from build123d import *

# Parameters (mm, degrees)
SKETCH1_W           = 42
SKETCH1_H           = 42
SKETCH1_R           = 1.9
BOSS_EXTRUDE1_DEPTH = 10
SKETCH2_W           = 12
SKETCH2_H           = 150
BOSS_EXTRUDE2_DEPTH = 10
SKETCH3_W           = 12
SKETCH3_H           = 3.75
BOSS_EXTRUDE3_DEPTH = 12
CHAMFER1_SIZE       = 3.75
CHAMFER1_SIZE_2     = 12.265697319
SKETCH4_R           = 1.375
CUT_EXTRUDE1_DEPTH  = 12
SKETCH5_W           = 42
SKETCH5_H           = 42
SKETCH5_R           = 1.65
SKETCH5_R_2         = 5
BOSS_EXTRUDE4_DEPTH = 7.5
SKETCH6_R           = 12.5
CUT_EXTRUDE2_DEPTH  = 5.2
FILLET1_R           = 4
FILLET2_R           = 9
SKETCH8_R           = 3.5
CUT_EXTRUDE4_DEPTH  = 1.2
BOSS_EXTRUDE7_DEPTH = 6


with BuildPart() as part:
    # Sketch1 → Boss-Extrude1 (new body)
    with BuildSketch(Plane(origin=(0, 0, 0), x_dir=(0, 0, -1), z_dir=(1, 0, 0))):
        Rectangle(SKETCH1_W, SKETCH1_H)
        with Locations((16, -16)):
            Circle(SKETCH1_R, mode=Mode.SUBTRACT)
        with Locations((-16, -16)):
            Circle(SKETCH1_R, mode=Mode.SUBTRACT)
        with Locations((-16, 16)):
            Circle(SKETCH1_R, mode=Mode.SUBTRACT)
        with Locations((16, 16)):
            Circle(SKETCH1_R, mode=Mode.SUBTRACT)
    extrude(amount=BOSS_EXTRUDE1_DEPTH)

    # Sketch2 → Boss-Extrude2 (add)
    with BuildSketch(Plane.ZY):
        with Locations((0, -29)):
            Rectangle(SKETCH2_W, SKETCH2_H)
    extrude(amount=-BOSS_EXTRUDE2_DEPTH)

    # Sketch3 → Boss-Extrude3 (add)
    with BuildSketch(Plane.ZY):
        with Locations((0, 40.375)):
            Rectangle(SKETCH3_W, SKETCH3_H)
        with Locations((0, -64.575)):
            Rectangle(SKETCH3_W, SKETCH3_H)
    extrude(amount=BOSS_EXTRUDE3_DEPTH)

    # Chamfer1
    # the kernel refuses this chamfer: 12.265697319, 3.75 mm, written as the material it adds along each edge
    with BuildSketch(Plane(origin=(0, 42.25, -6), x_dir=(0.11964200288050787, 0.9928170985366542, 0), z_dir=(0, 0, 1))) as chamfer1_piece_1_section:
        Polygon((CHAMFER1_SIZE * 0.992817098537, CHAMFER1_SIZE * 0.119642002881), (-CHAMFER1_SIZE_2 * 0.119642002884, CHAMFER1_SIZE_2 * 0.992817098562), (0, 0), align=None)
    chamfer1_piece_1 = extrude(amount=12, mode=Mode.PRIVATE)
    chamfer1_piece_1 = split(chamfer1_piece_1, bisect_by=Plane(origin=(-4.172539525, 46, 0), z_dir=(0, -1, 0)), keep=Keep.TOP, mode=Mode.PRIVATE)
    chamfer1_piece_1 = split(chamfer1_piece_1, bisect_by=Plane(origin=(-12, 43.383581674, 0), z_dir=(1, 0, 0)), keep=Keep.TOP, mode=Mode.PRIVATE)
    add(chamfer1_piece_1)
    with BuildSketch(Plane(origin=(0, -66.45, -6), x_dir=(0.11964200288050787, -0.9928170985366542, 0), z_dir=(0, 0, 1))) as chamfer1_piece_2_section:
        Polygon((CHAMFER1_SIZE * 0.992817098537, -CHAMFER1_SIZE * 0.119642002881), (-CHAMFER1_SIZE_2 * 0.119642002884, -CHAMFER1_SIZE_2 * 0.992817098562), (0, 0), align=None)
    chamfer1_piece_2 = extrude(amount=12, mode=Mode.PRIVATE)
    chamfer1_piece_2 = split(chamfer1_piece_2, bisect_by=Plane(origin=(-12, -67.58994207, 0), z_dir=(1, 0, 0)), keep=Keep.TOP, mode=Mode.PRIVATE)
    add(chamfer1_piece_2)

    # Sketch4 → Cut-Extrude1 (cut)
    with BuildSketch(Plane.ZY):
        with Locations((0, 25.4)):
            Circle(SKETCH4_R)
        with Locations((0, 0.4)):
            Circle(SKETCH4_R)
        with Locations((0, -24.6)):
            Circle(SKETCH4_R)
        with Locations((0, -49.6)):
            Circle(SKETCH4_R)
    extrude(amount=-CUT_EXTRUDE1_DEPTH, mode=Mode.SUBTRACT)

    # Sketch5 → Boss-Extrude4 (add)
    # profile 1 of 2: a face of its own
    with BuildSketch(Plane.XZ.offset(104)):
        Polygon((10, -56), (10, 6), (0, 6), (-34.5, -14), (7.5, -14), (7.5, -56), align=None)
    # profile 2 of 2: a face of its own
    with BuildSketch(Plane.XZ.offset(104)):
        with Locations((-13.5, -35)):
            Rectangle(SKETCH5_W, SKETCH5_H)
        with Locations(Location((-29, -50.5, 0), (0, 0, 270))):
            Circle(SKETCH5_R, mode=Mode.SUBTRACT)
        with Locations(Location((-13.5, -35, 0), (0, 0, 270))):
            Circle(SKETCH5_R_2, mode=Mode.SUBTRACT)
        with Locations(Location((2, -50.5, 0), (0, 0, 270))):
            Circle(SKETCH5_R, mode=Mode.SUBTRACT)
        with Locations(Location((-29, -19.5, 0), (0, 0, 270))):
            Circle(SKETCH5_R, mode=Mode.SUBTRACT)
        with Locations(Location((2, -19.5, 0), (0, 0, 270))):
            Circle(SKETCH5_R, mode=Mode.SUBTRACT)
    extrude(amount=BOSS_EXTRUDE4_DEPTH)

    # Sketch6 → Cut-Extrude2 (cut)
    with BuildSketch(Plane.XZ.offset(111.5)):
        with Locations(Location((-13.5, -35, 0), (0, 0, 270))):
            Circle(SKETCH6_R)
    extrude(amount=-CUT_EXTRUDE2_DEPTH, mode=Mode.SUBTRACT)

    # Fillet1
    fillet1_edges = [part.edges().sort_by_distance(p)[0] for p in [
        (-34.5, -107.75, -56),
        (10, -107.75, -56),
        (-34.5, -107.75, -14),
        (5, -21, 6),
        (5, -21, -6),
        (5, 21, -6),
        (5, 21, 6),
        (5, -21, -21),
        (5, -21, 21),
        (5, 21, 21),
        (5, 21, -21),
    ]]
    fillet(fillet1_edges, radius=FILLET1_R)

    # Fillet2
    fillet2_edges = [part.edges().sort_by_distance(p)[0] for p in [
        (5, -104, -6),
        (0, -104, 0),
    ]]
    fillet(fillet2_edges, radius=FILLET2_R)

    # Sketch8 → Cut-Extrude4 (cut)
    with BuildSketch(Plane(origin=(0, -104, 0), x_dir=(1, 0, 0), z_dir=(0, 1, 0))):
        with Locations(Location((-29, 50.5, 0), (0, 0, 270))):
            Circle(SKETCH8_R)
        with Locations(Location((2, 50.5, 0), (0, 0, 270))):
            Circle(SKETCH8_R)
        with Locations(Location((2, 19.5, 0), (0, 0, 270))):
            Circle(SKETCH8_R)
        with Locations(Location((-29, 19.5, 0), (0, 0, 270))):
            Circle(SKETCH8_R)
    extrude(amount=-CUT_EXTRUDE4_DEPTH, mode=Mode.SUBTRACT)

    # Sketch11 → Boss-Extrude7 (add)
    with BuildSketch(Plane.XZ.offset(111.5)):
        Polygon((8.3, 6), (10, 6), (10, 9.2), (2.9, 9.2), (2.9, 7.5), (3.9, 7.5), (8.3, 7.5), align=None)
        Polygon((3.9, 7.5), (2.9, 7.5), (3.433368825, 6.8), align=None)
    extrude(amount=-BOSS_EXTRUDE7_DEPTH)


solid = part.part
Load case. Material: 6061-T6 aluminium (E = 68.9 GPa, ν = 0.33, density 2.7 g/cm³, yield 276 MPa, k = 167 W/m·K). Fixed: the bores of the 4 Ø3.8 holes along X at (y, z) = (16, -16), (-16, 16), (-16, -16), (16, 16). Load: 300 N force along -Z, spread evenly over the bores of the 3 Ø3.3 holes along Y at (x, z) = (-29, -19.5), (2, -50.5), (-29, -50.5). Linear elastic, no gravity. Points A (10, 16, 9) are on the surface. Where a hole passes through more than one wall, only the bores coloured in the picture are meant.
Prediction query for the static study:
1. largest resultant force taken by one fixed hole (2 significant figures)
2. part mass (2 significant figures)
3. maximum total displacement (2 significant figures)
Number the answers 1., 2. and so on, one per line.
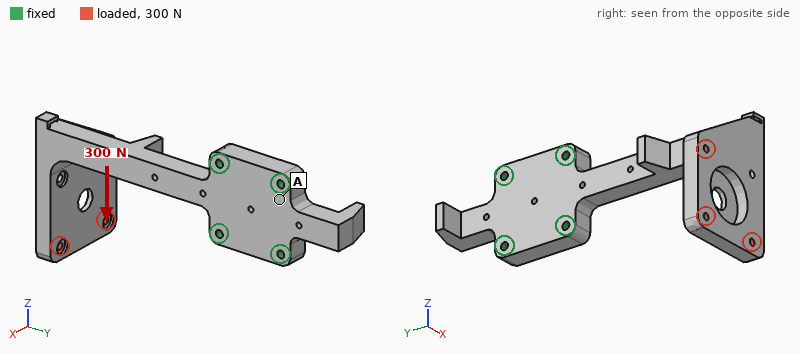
1. 810 N
2. 130 g
3. 1.5 mm
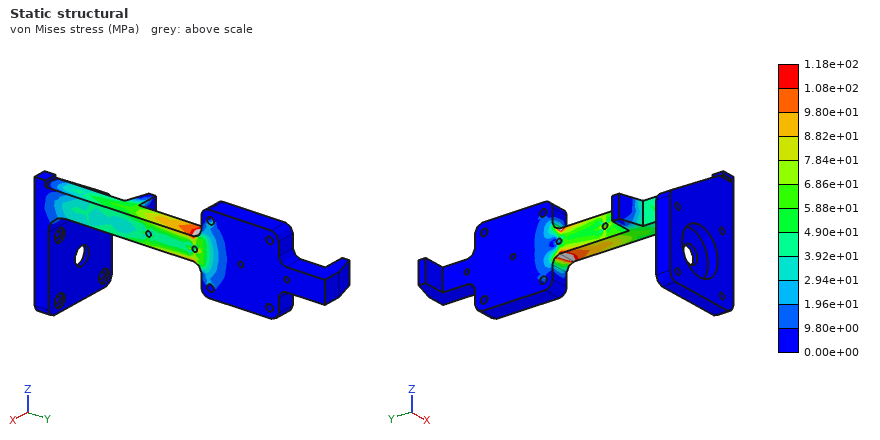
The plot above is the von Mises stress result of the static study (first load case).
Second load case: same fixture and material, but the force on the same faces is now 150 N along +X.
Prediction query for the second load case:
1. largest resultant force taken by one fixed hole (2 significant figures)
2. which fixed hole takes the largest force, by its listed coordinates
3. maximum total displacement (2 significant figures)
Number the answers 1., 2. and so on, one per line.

1. 450 N
2. (-16, -16)
3. 1.3 mm
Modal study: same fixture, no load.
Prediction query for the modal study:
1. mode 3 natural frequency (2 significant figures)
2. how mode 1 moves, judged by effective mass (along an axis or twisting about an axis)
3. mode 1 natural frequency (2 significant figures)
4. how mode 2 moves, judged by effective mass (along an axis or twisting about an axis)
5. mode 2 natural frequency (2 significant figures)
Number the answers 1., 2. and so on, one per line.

1. 890 Hz
2. along X
3. 310 Hz
4. along Z
5. 400 Hz
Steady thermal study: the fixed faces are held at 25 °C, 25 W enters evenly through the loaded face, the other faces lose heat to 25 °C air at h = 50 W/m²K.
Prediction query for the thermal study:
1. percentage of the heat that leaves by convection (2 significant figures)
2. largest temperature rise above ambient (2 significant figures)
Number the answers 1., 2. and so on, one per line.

1. 74 %
2. 55 K
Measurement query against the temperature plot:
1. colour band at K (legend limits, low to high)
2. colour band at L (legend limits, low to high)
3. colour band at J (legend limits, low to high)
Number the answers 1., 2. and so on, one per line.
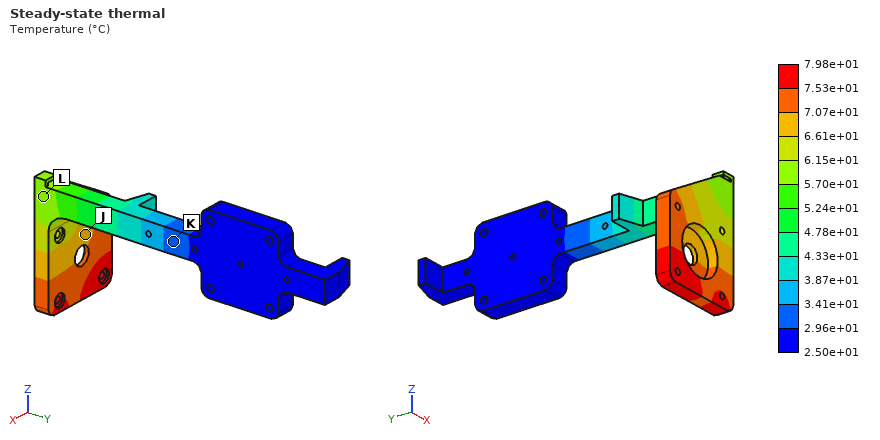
1. 2.96e+01 to 3.41e+01 °C
2. 5.70e+01 to 6.15e+01 °C
3. 6.61e+01 to 7.07e+01 °C
